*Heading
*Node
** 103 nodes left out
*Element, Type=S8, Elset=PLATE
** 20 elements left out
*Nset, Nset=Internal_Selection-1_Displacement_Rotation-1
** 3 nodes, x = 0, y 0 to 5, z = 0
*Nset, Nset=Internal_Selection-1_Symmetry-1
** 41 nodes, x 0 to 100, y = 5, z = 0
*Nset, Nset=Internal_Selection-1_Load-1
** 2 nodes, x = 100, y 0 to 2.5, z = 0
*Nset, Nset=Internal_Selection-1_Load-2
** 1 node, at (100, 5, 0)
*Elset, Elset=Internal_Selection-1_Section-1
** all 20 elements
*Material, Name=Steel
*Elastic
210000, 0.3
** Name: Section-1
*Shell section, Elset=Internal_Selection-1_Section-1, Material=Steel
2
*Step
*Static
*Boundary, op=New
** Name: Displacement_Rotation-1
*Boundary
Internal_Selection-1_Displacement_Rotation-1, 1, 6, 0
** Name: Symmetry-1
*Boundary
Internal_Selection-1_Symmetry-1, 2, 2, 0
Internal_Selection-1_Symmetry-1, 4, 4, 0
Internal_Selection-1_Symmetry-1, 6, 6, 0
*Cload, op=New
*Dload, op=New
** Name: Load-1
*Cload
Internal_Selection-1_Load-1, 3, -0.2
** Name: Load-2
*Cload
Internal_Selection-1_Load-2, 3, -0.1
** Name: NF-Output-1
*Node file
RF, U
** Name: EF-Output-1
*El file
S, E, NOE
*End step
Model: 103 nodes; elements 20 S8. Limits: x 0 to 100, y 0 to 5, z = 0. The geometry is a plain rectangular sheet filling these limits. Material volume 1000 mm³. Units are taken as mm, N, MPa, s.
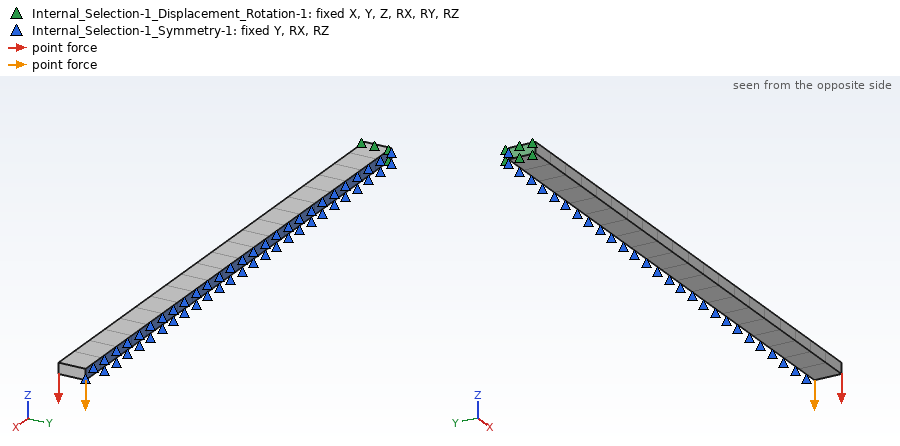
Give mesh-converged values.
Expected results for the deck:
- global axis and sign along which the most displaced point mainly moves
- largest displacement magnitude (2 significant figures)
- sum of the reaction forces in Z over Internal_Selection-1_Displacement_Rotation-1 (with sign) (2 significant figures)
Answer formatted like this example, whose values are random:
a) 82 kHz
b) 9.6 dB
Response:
a) -Z
b) 0.24 mm
c) 0.50 N
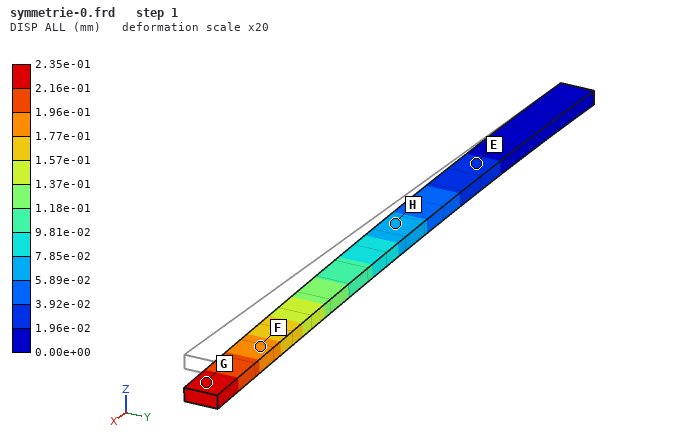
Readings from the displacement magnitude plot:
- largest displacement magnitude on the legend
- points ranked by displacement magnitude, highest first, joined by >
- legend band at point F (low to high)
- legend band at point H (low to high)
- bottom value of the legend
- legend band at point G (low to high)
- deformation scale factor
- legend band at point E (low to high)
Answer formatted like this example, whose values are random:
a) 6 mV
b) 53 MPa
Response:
a) 2.35e-01 mm
b) G > F > H > E
c) 1.77e-01 to 1.96e-01 mm
d) 5.89e-02 to 7.85e-02 mm
e) 0.00e+00 mm
f) 2.16e-01 to 2.35e-01 mm
g) 20
h) 1.96e-02 to 3.92e-02 mm
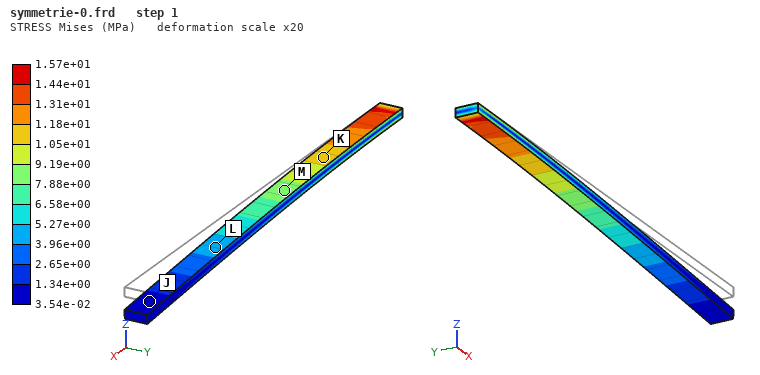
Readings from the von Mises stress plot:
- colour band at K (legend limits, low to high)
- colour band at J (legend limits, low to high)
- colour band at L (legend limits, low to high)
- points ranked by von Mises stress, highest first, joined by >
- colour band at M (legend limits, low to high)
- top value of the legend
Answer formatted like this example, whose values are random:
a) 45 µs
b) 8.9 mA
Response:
a) 1.05e+01 to 1.18e+01 MPa
b) 3.54e-02 to 1.34e+00 MPa
c) 3.96e+00 to 5.27e+00 MPa
d) K > M > L > J
e) 7.88e+00 to 9.19e+00 MPa
f) 1.57e+01 MPa
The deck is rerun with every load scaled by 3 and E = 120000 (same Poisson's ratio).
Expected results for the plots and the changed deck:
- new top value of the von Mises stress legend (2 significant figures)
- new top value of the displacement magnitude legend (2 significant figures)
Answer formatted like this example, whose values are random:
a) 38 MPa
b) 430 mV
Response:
a) 47 MPa
b) 1.2 mm
